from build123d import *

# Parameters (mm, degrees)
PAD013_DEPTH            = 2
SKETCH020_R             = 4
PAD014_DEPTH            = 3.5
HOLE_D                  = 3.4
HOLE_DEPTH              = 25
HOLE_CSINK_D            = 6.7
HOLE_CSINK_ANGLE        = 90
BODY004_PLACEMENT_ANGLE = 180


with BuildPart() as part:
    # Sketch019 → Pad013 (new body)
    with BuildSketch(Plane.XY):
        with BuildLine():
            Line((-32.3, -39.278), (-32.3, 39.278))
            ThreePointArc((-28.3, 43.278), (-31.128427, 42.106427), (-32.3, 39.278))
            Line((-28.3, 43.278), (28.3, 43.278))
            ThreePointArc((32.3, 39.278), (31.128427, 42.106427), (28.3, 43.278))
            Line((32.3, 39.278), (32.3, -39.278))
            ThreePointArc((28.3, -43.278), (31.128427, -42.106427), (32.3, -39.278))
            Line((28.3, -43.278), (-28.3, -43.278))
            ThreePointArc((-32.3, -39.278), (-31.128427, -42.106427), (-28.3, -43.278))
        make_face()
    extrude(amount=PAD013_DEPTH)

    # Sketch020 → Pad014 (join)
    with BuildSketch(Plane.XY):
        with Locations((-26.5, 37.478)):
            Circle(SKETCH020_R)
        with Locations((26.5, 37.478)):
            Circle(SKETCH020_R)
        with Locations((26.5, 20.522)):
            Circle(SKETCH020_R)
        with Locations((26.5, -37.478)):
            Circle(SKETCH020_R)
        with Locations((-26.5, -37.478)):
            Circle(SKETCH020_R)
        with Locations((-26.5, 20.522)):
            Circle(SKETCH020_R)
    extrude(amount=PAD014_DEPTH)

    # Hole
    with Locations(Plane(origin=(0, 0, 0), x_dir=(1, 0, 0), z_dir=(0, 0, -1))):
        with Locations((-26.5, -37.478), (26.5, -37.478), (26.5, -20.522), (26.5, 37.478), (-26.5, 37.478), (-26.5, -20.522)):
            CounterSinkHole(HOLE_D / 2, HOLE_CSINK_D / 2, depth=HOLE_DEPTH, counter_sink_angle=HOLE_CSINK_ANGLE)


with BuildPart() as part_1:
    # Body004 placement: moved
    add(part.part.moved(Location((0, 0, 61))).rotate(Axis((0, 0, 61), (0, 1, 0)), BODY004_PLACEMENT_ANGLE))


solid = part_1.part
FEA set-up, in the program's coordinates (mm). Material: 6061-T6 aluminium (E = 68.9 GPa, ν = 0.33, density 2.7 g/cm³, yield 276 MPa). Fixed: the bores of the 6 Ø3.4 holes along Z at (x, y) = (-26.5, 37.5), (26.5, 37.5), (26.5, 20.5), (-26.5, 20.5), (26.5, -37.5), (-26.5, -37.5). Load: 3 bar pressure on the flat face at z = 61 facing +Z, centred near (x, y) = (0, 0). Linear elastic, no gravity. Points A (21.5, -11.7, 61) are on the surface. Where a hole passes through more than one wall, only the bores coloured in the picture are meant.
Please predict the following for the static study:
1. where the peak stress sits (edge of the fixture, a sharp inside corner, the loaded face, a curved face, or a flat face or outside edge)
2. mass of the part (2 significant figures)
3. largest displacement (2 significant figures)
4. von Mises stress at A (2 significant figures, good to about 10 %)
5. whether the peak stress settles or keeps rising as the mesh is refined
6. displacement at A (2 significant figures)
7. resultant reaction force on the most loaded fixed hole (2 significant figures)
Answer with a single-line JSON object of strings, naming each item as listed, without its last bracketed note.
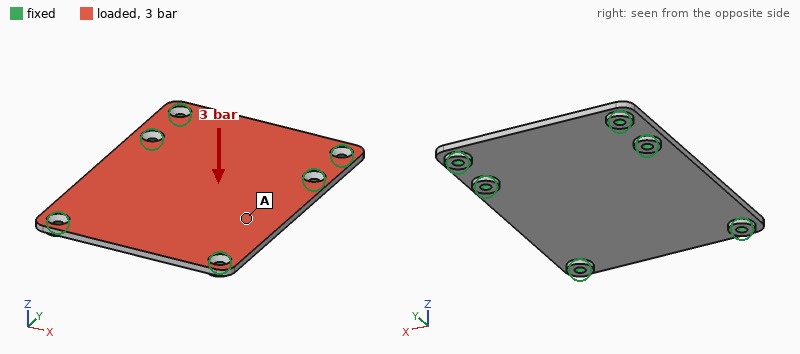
{"where the peak stress sits": "edge of the fixture", "mass of the part": "31 g", "largest displacement": "0.35 mm", "von Mises stress at A": "71 MPa", "whether the peak stress settles or keeps rising as the mesh is refined": "keeps rising", "displacement at A": "0.25 mm", "resultant reaction force on the most loaded fixed hole": "680 N"}
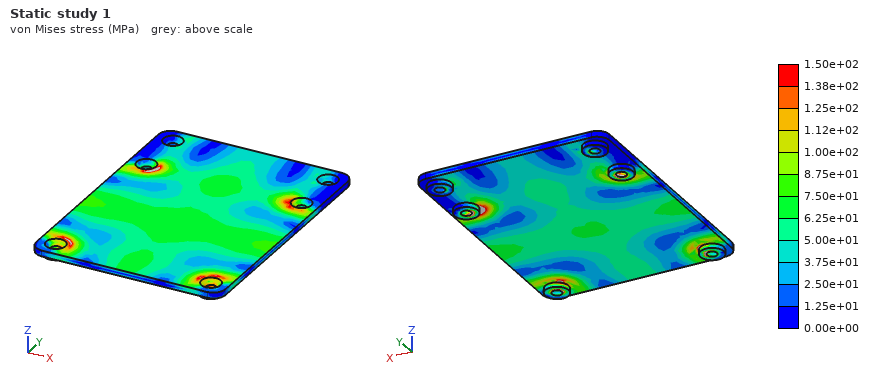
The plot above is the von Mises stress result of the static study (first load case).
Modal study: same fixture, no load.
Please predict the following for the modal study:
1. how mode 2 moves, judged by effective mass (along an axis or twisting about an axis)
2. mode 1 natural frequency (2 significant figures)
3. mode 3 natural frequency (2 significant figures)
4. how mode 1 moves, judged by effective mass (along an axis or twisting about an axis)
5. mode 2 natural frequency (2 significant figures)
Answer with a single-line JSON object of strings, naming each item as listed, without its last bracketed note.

{"how mode 2 moves, judged by effective mass": "twisting about Y", "mode 1 natural frequency": "2500 Hz", "mode 3 natural frequency": "4200 Hz", "how mode 1 moves, judged by effective mass": "along Z", "mode 2 natural frequency": "3800 Hz"}
